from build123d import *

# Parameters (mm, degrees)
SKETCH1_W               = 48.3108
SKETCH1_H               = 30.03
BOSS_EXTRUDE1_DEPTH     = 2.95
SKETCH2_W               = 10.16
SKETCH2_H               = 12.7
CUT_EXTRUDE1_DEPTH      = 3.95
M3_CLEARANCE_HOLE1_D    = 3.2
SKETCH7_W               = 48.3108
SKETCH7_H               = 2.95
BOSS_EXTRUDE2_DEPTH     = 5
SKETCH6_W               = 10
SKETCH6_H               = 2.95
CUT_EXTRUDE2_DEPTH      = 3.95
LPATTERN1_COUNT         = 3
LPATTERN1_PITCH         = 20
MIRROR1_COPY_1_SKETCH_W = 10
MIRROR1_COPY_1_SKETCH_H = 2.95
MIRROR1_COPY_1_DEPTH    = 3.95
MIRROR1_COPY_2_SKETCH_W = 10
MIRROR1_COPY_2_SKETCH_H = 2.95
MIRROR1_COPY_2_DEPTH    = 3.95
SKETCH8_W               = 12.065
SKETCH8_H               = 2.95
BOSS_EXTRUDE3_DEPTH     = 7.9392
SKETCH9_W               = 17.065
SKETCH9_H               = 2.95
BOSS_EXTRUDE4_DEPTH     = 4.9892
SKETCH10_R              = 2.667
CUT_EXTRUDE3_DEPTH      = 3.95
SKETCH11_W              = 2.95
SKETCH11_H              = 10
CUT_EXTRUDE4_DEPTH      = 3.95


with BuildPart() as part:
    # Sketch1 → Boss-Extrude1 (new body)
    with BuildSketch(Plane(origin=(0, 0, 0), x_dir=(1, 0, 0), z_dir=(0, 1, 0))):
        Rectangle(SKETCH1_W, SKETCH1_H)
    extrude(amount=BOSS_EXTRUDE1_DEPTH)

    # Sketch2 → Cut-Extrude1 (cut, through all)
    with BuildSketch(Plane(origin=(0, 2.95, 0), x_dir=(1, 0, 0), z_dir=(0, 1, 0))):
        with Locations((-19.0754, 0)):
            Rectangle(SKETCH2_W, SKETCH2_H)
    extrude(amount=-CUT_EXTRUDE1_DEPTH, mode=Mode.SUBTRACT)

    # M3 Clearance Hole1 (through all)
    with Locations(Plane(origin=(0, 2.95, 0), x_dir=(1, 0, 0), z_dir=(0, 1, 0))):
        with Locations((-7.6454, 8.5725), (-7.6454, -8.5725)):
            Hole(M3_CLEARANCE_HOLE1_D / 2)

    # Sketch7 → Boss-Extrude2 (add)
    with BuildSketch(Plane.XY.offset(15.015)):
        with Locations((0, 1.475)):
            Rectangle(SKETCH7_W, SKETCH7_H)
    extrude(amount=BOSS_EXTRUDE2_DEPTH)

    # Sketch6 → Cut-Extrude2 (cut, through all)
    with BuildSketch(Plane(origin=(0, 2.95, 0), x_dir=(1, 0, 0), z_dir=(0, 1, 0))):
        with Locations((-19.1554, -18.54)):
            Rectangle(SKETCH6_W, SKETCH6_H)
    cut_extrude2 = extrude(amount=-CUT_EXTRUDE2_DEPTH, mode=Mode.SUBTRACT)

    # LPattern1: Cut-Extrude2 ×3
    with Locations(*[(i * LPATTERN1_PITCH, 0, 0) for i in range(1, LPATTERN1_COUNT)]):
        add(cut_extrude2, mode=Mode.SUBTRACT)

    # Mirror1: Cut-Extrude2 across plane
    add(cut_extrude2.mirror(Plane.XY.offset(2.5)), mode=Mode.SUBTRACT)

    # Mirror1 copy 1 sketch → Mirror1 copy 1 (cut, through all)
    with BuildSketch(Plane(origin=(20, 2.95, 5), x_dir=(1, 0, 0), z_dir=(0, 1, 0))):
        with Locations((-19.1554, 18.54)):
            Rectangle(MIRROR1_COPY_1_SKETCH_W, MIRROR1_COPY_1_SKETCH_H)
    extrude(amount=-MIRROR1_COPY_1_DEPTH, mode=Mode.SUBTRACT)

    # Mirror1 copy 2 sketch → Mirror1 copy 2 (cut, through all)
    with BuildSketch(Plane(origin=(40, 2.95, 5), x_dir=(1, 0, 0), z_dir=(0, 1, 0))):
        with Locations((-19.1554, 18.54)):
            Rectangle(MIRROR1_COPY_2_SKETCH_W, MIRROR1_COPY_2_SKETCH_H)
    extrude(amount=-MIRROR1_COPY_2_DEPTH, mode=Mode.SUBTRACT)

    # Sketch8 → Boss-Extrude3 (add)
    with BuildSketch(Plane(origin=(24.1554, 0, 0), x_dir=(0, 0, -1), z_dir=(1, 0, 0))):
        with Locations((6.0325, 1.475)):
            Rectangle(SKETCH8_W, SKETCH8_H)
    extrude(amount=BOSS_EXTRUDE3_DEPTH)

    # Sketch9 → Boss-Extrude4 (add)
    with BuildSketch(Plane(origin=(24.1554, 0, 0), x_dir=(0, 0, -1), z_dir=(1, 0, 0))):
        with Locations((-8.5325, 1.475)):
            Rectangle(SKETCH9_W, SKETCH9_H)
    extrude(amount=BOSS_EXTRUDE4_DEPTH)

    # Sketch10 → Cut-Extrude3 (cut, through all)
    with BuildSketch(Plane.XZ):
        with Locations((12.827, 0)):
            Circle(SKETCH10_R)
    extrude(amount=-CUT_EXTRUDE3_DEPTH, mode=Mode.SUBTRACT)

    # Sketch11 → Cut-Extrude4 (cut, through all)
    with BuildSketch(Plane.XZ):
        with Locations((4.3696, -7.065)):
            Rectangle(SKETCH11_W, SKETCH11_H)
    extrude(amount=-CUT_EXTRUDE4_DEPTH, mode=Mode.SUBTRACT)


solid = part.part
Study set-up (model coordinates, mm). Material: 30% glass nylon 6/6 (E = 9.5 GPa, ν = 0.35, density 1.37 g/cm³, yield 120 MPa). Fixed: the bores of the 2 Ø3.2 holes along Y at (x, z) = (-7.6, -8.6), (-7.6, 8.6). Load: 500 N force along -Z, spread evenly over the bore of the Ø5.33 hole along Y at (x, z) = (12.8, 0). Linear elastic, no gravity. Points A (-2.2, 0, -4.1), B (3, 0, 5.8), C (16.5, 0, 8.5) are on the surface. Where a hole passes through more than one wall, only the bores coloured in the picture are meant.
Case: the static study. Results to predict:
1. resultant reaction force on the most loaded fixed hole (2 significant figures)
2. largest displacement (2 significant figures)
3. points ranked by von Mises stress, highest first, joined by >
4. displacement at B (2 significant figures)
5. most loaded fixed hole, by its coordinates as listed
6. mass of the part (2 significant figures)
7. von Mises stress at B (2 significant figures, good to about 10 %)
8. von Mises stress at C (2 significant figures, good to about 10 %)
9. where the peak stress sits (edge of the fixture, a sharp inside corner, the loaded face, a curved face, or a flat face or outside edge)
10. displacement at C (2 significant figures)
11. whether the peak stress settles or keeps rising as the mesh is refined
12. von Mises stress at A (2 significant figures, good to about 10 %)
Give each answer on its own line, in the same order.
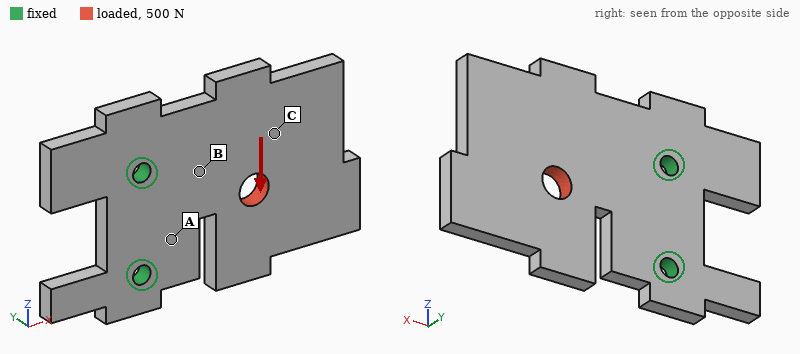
620 N
0.29 mm
A > B > C
0.046 mm
(-7.6, -8.6)
6.1 g
19 MPa
7.8 MPa
a sharp inside corner
0.15 mm
keeps rising
32 MPa
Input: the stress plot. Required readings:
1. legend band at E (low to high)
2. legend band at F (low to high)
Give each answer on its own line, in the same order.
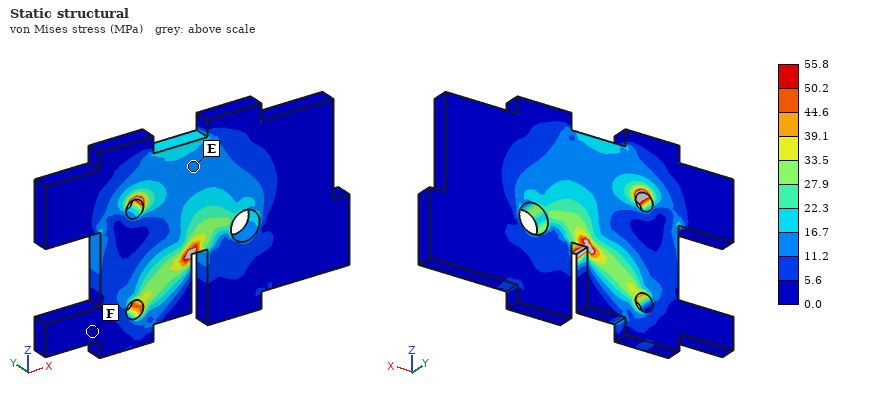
11.2 to 16.7 MPa
0.0 to 5.6 MPa
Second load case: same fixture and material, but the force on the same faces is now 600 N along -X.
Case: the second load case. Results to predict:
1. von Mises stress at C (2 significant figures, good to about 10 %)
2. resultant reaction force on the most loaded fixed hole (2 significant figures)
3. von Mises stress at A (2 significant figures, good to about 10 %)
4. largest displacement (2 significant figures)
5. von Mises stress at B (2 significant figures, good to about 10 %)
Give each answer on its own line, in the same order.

6.0 MPa
330 N
17 MPa
0.17 mm
9.9 MPa
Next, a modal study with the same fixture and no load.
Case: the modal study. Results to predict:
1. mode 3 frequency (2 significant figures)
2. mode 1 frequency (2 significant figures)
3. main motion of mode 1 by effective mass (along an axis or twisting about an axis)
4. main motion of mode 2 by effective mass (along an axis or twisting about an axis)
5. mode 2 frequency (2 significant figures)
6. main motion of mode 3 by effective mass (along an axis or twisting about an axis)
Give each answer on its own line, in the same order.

3600 Hz
760 Hz
along Y
twisting about X
1800 Hz
along Z
